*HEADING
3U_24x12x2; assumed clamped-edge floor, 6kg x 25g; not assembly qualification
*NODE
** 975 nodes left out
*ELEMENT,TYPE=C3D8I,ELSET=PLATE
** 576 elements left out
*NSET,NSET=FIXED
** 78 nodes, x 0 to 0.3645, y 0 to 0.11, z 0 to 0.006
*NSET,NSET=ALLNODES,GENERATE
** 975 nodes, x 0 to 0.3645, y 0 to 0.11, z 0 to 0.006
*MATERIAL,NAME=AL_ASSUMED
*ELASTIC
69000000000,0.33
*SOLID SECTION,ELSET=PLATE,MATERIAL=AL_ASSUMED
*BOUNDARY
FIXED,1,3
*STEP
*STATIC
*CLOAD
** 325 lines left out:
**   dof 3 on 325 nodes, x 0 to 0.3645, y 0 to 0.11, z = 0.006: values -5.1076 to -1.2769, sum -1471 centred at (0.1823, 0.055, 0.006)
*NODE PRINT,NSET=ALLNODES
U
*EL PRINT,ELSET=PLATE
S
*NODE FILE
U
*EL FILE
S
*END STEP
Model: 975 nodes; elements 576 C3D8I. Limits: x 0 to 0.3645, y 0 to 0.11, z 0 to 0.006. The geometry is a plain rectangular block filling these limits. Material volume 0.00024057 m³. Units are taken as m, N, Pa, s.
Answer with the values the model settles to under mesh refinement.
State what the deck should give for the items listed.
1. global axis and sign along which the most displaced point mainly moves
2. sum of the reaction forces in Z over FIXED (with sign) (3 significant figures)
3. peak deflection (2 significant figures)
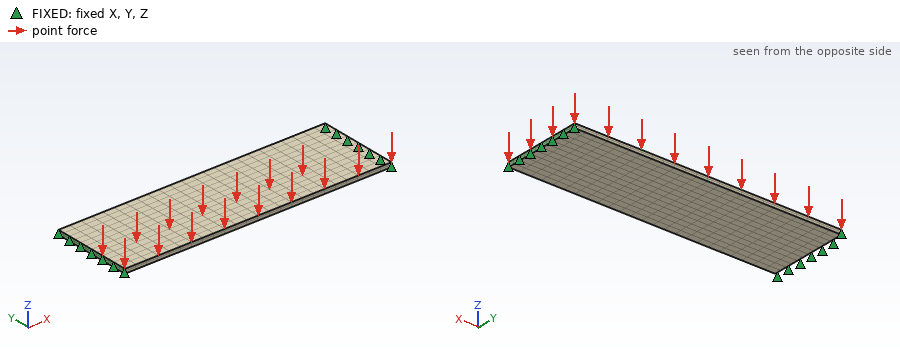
-Z
1470 N
0.0013 m
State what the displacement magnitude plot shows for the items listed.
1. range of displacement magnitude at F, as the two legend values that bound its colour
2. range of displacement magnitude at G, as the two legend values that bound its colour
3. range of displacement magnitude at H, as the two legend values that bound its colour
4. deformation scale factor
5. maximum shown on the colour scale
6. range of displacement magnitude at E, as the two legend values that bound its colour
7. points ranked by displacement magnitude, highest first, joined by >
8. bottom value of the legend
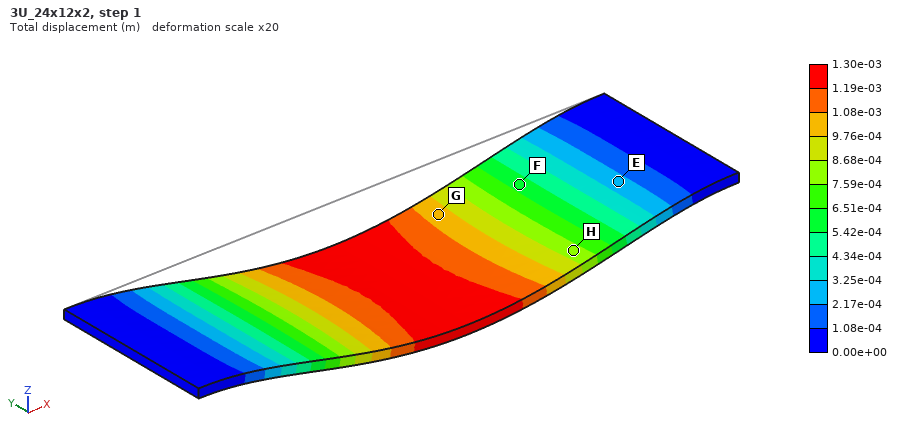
5.42e-04 to 6.51e-04 m
9.76e-04 to 1.08e-03 m
7.59e-04 to 8.68e-04 m
20
1.30e-03 m
2.17e-04 to 3.25e-04 m
G > H > F > E
0.00e+00 m
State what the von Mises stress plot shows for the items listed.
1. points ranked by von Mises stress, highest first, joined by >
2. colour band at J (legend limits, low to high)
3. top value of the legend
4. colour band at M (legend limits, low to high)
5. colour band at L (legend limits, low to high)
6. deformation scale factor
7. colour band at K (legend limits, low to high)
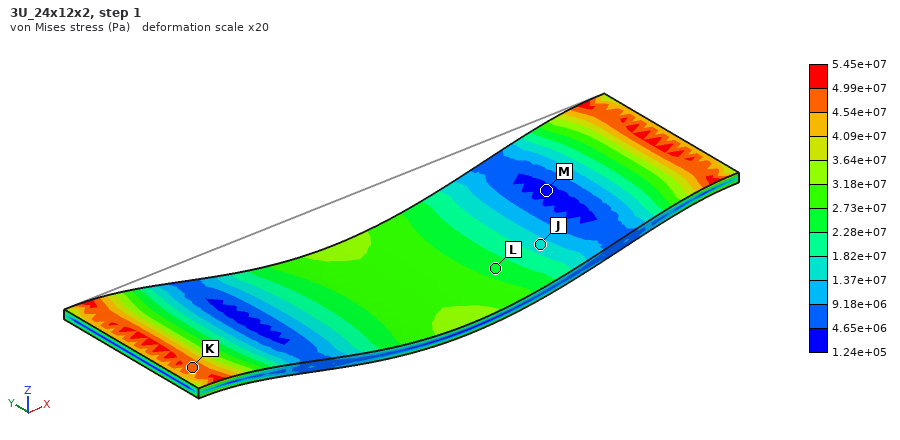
K > L > J > M
1.37e+07 to 1.82e+07 Pa
5.45e+07 Pa
1.24e+05 to 4.65e+06 Pa
2.28e+07 to 2.73e+07 Pa
20
4.54e+07 to 4.99e+07 Pa
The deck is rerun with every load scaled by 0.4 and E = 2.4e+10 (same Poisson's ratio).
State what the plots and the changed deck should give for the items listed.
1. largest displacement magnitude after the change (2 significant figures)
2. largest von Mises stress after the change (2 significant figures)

0.0015 m
2.2e+07 Pa
